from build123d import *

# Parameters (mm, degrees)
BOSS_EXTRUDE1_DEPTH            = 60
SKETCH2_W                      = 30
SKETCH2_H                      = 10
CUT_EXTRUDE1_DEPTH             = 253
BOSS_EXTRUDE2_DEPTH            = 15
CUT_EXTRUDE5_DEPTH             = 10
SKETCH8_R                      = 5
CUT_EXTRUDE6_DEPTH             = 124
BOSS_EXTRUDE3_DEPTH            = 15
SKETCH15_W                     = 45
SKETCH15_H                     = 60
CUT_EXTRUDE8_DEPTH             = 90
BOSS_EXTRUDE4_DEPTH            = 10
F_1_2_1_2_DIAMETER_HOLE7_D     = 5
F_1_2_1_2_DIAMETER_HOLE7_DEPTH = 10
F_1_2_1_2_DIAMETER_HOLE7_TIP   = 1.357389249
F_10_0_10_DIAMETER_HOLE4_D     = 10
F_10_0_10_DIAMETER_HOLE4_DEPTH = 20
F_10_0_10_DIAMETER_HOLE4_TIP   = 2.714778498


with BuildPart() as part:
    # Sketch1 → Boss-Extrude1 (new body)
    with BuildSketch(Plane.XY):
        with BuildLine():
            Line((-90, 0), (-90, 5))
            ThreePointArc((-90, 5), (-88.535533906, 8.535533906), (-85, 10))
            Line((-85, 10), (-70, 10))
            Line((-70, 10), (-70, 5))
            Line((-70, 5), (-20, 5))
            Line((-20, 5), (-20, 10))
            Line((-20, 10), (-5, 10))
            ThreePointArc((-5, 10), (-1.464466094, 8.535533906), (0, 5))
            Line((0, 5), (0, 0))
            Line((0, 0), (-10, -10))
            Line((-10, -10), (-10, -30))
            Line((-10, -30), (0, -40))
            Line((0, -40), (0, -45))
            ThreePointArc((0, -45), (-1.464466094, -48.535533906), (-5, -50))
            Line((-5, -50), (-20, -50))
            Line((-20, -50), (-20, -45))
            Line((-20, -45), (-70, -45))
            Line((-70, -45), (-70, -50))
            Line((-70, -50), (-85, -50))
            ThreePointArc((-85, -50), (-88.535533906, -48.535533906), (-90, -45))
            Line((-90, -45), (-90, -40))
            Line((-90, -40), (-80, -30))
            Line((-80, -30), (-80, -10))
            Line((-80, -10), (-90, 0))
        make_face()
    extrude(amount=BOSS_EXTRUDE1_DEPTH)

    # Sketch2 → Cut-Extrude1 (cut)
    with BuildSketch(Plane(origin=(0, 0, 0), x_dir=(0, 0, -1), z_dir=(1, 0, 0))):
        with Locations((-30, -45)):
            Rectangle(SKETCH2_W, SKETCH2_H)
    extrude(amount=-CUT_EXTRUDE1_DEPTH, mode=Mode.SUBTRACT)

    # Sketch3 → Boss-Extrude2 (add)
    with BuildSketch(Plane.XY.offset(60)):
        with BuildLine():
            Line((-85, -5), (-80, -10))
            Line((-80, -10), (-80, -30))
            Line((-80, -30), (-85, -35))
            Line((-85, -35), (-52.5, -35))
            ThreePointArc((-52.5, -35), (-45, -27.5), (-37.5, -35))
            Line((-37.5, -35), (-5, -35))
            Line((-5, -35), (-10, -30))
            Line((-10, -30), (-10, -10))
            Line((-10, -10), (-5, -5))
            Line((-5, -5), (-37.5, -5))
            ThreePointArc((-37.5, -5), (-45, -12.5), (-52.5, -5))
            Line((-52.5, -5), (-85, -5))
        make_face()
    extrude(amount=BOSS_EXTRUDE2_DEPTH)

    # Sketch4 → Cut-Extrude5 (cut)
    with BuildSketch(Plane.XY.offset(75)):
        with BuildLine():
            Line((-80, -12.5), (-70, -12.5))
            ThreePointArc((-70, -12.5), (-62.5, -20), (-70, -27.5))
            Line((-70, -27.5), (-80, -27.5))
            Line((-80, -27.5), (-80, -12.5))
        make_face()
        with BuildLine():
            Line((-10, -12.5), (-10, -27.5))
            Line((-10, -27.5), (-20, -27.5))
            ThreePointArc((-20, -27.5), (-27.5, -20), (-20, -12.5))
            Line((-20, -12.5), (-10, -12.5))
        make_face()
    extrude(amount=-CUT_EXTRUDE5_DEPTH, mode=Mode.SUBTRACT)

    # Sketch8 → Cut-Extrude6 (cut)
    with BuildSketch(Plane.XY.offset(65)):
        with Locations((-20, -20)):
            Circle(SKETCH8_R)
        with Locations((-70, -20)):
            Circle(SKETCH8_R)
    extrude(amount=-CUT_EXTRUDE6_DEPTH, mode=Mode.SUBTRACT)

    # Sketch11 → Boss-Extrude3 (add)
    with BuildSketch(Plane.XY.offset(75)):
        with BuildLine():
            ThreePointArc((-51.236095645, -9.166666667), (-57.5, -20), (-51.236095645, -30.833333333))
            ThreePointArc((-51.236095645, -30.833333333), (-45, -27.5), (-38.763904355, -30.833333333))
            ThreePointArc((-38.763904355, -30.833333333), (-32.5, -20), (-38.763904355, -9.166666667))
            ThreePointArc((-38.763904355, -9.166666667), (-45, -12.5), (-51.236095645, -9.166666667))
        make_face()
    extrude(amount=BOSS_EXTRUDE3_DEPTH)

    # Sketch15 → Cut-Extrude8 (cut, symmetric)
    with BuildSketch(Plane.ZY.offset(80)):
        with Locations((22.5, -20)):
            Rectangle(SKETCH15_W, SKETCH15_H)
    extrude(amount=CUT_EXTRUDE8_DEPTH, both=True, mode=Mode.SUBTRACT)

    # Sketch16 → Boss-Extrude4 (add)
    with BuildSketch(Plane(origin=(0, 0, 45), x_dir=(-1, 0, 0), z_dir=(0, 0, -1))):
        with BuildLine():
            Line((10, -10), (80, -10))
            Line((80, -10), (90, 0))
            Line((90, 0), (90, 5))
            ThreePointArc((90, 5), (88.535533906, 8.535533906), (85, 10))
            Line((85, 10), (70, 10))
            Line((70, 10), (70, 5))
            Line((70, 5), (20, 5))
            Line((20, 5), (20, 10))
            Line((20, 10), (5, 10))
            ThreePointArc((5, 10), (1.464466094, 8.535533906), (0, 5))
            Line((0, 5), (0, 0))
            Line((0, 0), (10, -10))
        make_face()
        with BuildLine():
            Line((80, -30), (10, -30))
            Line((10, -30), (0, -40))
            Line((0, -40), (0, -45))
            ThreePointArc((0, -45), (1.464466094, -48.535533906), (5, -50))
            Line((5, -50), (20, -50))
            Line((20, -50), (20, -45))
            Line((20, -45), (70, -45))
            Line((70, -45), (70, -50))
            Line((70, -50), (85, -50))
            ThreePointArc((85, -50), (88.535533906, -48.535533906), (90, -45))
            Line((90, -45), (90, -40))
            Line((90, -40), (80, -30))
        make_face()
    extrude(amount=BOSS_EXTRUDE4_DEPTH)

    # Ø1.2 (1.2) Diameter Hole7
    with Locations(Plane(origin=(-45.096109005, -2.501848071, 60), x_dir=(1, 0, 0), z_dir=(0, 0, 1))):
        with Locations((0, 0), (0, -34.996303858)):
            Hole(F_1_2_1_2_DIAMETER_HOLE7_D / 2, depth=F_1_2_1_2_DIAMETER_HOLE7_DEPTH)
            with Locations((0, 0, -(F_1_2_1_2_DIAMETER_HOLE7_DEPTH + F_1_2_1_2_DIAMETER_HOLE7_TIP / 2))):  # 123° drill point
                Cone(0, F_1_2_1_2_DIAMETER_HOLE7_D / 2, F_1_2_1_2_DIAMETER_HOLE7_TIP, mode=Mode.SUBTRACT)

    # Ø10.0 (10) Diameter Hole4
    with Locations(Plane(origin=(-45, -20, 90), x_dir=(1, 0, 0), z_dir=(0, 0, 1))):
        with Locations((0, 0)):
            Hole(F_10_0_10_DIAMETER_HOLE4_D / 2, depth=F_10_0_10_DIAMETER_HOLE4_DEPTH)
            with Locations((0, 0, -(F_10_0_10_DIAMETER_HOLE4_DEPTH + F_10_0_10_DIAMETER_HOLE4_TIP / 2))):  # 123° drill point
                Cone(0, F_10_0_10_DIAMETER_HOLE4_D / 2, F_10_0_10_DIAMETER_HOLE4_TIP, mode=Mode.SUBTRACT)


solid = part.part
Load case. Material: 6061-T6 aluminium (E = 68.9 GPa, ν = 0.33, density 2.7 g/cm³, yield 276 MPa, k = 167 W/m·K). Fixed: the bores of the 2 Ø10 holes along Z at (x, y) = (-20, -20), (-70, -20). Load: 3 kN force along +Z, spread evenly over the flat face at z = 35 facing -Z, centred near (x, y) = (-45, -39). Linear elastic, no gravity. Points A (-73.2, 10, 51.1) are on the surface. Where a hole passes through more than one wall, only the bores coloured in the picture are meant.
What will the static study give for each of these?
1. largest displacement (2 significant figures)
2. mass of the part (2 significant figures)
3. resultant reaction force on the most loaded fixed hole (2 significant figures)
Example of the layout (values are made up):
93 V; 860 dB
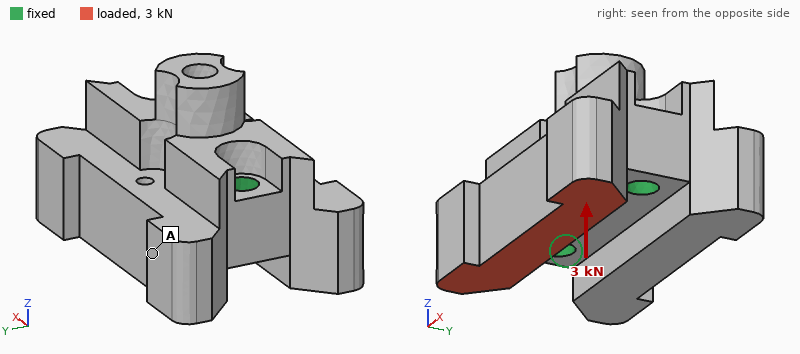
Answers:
8.9 µm; 320 g; 1.5 kN
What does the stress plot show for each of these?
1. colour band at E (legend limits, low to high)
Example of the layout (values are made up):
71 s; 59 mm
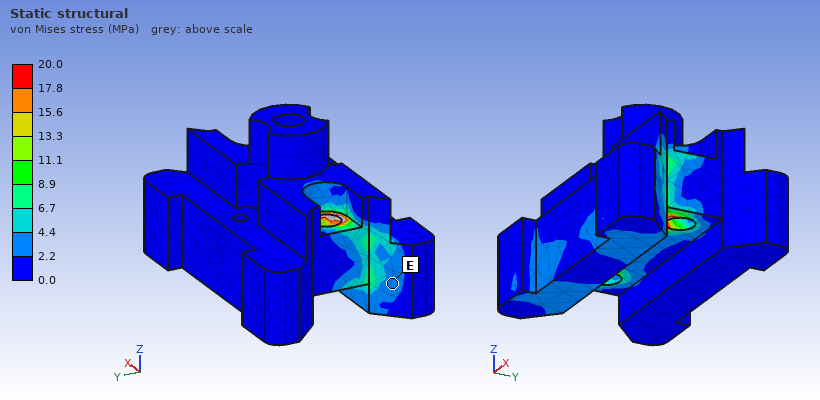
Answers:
2.2 to 4.4 MPa
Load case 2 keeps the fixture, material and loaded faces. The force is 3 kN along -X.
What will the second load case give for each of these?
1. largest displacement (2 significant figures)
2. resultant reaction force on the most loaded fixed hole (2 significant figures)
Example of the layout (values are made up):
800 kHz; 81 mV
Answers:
8.6 µm; 2.0 kN
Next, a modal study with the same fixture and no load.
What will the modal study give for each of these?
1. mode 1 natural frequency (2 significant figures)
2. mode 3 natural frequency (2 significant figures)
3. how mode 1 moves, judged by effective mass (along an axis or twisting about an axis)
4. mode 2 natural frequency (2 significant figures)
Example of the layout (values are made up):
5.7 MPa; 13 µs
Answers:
9700 Hz; 13 kHz; twisting about X; 12 kHz
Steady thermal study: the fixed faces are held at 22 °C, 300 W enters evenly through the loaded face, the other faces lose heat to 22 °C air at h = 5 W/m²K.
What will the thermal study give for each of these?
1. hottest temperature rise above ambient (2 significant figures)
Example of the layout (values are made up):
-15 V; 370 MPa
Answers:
44 K
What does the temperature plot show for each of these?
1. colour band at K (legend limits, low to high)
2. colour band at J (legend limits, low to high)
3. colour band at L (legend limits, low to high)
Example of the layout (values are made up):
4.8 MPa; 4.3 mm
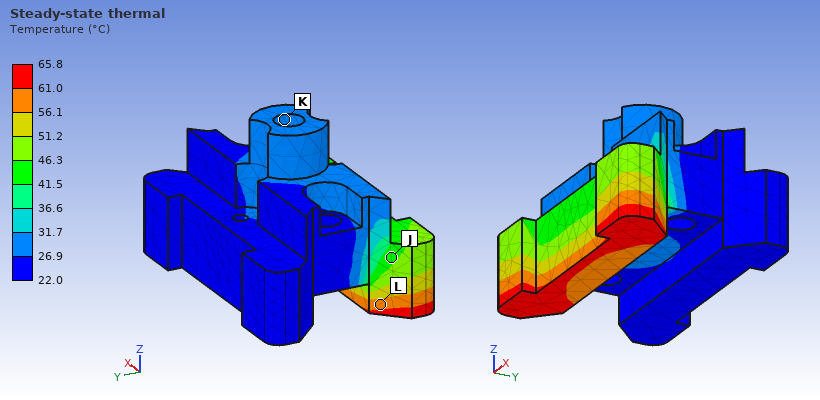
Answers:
26.9 to 31.7 °C; 41.5 to 46.3 °C; 56.1 to 61.0 °C
